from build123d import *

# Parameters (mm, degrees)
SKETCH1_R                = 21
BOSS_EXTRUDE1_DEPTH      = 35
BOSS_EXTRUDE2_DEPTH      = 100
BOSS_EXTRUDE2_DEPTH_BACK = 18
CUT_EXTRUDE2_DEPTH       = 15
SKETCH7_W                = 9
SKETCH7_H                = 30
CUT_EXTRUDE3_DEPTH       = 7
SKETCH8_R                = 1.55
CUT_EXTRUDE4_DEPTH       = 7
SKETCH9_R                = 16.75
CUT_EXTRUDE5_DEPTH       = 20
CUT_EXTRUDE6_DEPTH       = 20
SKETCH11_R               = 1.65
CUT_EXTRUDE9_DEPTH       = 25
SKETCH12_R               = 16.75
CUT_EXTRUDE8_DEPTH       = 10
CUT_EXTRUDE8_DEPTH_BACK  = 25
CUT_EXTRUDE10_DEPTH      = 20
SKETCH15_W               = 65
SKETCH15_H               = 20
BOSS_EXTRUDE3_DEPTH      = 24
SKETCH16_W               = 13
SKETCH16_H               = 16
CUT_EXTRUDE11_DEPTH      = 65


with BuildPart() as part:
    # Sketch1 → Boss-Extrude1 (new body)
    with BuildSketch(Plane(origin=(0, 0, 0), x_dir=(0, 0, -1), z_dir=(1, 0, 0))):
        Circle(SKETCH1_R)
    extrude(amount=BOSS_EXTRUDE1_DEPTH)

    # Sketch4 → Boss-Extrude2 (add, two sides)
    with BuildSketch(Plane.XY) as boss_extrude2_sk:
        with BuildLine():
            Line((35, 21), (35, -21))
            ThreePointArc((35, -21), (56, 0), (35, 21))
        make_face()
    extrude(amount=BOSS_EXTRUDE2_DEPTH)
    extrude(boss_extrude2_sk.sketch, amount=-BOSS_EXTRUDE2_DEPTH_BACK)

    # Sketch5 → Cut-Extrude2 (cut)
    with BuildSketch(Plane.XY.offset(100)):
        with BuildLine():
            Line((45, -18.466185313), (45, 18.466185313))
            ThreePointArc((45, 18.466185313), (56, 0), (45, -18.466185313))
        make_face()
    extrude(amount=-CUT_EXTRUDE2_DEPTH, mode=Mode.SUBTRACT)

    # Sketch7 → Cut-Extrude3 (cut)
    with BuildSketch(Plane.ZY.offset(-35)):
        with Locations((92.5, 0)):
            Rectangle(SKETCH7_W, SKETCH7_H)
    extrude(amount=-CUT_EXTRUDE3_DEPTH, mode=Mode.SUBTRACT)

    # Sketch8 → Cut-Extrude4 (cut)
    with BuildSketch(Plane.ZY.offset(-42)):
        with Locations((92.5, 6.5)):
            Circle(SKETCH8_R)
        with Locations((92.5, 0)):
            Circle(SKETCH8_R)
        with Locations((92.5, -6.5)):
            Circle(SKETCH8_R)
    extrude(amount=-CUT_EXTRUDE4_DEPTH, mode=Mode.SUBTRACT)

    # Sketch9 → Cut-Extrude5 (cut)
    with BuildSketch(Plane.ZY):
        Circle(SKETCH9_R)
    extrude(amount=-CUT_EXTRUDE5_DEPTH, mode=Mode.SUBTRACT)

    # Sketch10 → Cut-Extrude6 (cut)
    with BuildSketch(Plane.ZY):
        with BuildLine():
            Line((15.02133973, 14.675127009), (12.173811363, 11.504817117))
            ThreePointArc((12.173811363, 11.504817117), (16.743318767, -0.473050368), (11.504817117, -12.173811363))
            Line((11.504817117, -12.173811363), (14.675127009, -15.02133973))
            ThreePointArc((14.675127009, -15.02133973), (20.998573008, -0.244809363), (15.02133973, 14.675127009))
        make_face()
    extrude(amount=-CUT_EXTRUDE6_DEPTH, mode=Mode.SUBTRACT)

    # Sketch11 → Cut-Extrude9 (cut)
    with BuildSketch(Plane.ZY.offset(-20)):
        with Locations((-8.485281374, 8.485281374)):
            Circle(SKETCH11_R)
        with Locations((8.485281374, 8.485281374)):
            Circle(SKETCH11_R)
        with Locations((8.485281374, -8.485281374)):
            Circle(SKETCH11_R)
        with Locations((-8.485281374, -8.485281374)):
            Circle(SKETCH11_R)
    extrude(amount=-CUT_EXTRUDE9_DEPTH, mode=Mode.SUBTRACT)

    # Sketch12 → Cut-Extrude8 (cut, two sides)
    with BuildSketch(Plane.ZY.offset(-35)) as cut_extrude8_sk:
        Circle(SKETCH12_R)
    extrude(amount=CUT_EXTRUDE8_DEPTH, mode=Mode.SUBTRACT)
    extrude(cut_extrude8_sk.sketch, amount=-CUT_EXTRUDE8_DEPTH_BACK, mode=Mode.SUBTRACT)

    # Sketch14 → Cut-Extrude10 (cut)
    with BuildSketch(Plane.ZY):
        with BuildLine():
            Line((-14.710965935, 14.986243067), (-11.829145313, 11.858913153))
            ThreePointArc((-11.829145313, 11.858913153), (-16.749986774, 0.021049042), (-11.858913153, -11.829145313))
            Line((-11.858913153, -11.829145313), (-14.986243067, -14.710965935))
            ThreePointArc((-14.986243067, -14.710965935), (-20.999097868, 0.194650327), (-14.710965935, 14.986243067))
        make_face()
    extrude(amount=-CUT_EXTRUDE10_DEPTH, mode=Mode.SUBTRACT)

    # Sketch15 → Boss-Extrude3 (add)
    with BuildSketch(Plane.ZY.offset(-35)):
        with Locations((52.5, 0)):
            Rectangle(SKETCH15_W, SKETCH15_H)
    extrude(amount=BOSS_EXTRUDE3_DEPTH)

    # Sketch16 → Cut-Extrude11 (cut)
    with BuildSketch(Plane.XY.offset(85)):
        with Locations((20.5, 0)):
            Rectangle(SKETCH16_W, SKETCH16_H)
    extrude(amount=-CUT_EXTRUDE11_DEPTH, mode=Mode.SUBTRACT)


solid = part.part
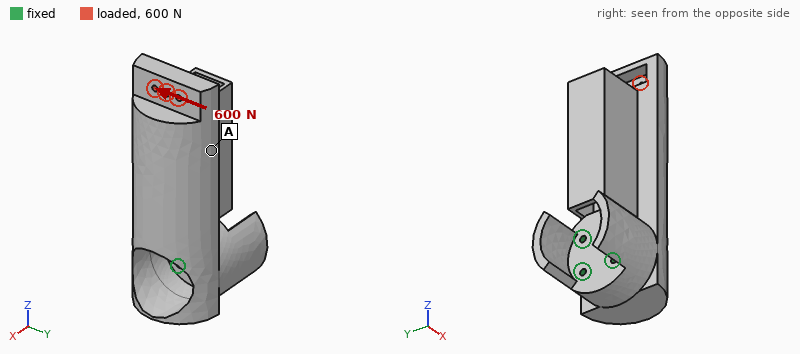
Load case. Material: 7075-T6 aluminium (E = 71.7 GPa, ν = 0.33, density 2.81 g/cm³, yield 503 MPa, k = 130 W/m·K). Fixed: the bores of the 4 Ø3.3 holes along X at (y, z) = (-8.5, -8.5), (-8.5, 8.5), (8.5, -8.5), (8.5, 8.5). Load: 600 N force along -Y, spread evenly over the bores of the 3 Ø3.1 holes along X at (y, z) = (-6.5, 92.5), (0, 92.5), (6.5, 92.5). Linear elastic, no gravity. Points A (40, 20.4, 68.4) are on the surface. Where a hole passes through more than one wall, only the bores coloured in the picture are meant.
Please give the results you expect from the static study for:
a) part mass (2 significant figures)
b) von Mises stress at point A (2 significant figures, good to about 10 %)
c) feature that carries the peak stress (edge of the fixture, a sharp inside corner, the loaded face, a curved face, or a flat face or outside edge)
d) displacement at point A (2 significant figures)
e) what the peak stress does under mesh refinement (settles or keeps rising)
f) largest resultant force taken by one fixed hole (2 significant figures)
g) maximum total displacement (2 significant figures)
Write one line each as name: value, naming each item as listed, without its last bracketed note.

part mass: 260 g
von Mises stress at point A: 3.8 MPa
feature that carries the peak stress: edge of the fixture
displacement at point A: 0.062 mm
what the peak stress does under mesh refinement: keeps rising
largest resultant force taken by one fixed hole: 1.3 kN
maximum total displacement: 0.10 mm
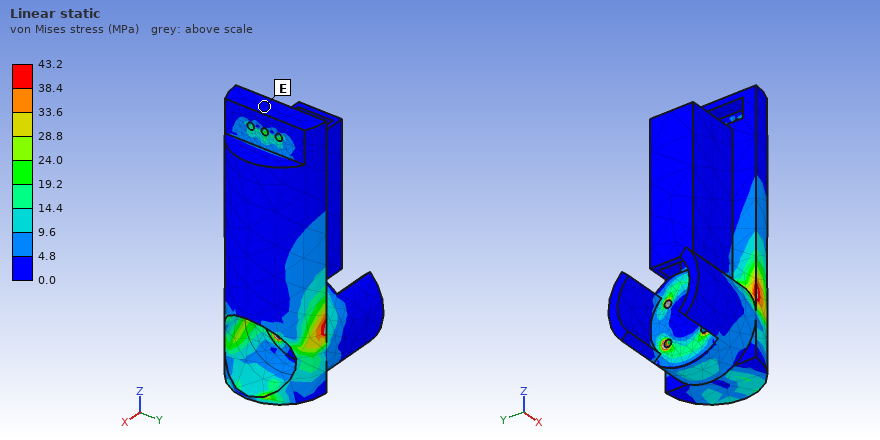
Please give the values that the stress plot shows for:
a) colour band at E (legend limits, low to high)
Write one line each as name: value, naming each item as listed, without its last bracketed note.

colour band at E: 0.0 to 4.8 MPa
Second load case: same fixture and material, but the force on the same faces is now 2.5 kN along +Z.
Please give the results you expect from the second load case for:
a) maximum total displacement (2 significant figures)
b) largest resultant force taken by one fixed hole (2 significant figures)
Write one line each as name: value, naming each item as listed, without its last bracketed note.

maximum total displacement: 0.15 mm
largest resultant force taken by one fixed hole: 1.3 kN
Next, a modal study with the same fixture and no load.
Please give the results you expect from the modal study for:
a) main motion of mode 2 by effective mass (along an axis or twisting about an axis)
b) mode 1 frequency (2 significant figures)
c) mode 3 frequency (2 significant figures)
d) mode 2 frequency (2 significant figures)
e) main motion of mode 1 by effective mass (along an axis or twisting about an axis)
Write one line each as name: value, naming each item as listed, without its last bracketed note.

main motion of mode 2 by effective mass: along Y
mode 1 frequency: 1100 Hz
mode 3 frequency: 3500 Hz
mode 2 frequency: 1600 Hz
main motion of mode 1 by effective mass: along X
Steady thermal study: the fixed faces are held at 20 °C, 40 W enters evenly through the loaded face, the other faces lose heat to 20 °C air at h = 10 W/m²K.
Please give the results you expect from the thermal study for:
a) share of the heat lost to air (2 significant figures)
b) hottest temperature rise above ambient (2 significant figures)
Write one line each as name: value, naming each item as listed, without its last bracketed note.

share of the heat lost to air: 16 %
hottest temperature rise above ambient: 67 K
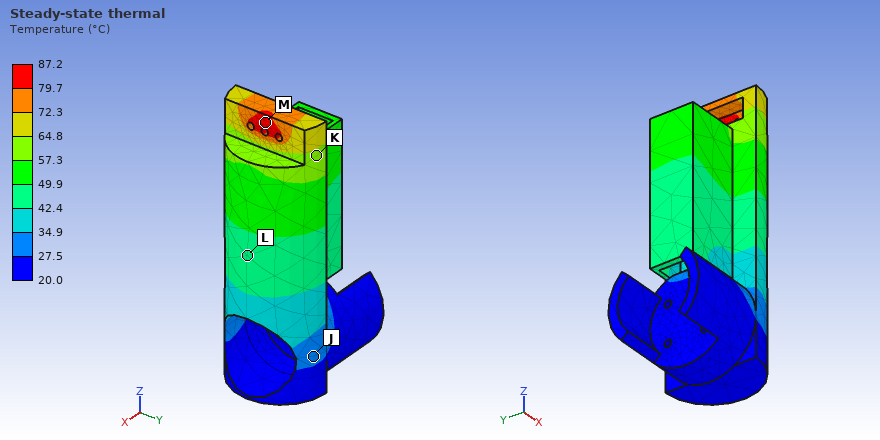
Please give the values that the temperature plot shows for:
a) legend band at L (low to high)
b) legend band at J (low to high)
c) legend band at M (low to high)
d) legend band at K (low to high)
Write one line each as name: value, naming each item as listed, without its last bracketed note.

legend band at L: 42.4 to 49.9 °C
legend band at J: 27.5 to 34.9 °C
legend band at M: 79.7 to 87.2 °C
legend band at K: 57.3 to 64.8 °C
